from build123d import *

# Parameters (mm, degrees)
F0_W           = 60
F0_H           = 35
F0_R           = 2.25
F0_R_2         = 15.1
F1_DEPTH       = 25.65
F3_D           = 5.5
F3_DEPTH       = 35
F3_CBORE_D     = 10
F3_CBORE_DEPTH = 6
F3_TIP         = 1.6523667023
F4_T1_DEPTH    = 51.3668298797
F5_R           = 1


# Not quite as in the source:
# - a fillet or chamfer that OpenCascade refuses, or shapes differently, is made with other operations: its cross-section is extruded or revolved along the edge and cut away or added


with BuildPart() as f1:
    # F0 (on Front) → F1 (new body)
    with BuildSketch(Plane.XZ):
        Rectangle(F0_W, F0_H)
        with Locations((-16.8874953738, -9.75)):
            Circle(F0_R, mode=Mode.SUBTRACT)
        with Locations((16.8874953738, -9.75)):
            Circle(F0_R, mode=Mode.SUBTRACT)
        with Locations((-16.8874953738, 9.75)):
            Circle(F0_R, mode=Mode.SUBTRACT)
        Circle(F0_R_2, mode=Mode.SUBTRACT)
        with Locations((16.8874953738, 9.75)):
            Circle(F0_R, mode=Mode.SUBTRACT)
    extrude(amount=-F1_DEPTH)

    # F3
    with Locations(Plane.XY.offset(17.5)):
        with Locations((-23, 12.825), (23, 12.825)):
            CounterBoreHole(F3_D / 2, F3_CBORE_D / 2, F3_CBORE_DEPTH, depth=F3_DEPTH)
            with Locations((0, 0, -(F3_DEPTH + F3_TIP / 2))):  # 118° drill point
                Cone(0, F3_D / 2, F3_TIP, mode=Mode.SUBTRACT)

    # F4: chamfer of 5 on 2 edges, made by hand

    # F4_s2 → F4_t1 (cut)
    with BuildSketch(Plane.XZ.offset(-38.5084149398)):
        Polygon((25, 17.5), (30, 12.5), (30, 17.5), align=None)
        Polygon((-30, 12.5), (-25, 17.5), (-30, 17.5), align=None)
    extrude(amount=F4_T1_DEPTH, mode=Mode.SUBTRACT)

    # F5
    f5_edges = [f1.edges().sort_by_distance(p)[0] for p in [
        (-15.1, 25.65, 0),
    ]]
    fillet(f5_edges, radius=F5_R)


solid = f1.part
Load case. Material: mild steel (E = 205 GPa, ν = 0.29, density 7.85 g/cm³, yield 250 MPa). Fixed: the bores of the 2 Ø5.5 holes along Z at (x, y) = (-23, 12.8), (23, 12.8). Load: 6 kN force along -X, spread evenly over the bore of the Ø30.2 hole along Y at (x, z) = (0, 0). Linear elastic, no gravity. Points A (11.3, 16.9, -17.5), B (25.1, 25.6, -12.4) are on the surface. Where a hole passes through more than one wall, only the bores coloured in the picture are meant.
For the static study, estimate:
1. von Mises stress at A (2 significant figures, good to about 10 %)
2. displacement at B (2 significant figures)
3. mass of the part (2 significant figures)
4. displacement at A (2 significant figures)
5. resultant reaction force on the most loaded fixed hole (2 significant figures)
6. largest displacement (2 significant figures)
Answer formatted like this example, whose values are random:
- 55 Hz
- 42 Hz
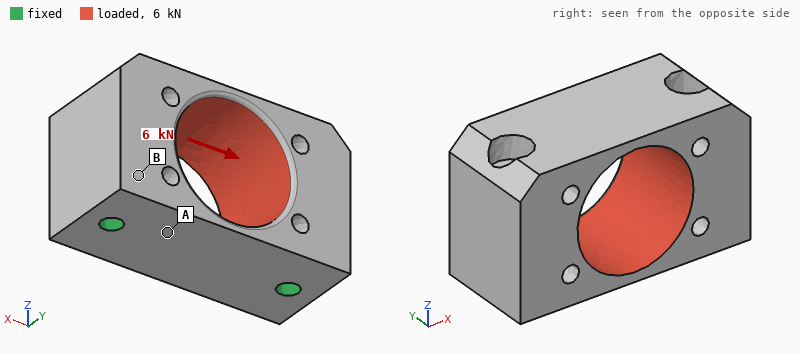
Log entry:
- 6.1 MPa
- 0.28 µm
- 240 g
- 0.41 µm
- 3.0 kN
- 1.6 µm
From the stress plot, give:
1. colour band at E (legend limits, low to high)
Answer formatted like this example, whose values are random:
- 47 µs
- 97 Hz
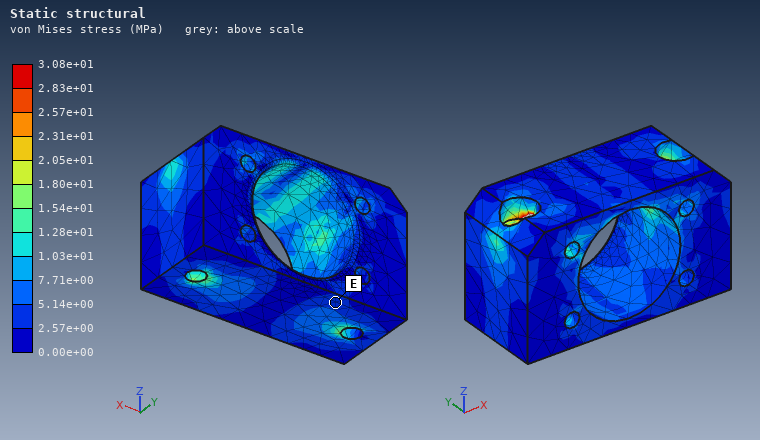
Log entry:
- 2.57e+00 to 5.14e+00 MPa
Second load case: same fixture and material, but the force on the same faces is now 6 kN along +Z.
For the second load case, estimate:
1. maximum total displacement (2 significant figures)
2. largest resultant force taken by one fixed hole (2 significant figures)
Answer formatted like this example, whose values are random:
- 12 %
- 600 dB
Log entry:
- 4.0 µm
- 3.0 kN
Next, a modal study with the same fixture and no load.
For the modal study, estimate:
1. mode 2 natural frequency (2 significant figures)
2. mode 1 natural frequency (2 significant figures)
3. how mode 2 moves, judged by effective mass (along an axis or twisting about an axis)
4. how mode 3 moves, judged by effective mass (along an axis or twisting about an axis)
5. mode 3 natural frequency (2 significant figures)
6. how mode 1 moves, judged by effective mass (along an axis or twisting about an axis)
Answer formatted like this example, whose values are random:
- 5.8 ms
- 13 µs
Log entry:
- 25 kHz
- 21 kHz
- along X
- twisting about X
- 27 kHz
- along Y
